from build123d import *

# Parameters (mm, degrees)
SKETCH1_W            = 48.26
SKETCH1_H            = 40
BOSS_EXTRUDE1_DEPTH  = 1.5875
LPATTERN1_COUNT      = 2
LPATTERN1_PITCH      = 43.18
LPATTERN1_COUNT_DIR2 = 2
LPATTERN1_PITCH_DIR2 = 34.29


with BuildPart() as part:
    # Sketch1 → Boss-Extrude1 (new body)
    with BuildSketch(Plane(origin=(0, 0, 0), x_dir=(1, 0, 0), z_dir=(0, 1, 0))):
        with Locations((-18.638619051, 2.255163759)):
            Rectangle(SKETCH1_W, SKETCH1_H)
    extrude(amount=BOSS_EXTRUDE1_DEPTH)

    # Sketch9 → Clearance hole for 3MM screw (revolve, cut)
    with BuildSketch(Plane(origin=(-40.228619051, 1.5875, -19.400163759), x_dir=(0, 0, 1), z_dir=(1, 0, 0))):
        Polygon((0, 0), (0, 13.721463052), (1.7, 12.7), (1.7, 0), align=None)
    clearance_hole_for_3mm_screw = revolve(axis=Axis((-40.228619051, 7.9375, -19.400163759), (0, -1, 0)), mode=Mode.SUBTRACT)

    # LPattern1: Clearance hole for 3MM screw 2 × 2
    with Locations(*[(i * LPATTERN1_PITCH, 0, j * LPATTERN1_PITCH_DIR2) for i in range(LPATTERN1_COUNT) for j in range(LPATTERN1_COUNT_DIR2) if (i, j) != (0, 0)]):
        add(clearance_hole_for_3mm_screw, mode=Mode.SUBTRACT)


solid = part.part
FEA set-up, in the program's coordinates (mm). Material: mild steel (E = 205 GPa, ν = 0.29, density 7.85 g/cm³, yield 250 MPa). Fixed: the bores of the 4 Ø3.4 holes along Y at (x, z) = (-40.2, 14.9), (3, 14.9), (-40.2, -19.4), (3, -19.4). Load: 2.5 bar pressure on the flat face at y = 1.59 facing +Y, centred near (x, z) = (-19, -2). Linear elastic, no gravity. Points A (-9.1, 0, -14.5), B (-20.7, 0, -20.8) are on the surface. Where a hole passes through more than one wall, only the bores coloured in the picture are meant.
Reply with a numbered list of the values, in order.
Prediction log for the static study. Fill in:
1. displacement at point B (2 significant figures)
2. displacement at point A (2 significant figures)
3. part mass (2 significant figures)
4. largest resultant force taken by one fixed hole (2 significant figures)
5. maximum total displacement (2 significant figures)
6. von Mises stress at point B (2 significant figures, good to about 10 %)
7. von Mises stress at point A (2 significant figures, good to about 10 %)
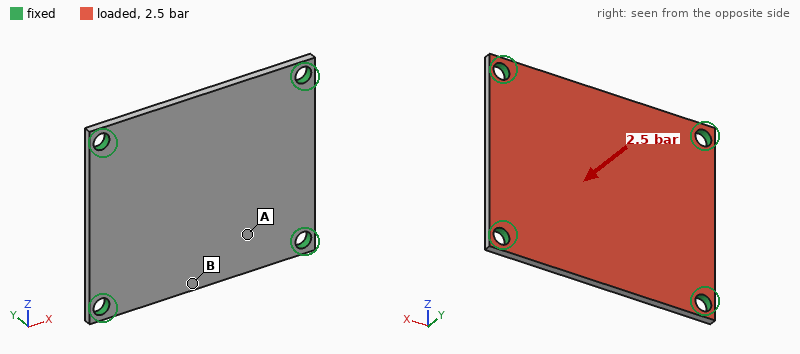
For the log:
1. 38 µm
2. 32 µm
3. 24 g
4. 120 N
5. 54 µm
6. 57 MPa
7. 28 MPa
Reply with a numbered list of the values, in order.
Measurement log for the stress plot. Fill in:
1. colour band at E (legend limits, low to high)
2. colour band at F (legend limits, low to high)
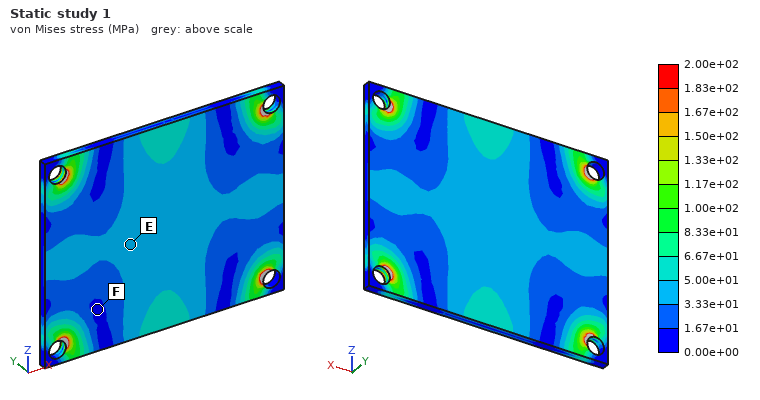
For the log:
1. 3.33e+01 to 5.00e+01 MPa
2. 0.00e+00 to 1.67e+01 MPa
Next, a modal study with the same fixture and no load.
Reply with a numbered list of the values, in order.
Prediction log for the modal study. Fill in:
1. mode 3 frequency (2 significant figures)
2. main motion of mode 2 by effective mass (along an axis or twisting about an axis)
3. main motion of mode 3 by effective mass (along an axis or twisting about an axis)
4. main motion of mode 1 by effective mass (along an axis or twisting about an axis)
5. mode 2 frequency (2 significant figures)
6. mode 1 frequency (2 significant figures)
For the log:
1. 7700 Hz
2. twisting about X
3. twisting about Z
4. along Y
5. 5800 Hz
6. 3700 Hz
